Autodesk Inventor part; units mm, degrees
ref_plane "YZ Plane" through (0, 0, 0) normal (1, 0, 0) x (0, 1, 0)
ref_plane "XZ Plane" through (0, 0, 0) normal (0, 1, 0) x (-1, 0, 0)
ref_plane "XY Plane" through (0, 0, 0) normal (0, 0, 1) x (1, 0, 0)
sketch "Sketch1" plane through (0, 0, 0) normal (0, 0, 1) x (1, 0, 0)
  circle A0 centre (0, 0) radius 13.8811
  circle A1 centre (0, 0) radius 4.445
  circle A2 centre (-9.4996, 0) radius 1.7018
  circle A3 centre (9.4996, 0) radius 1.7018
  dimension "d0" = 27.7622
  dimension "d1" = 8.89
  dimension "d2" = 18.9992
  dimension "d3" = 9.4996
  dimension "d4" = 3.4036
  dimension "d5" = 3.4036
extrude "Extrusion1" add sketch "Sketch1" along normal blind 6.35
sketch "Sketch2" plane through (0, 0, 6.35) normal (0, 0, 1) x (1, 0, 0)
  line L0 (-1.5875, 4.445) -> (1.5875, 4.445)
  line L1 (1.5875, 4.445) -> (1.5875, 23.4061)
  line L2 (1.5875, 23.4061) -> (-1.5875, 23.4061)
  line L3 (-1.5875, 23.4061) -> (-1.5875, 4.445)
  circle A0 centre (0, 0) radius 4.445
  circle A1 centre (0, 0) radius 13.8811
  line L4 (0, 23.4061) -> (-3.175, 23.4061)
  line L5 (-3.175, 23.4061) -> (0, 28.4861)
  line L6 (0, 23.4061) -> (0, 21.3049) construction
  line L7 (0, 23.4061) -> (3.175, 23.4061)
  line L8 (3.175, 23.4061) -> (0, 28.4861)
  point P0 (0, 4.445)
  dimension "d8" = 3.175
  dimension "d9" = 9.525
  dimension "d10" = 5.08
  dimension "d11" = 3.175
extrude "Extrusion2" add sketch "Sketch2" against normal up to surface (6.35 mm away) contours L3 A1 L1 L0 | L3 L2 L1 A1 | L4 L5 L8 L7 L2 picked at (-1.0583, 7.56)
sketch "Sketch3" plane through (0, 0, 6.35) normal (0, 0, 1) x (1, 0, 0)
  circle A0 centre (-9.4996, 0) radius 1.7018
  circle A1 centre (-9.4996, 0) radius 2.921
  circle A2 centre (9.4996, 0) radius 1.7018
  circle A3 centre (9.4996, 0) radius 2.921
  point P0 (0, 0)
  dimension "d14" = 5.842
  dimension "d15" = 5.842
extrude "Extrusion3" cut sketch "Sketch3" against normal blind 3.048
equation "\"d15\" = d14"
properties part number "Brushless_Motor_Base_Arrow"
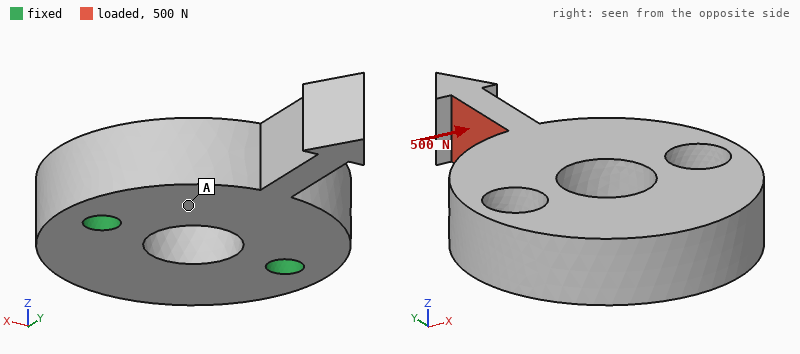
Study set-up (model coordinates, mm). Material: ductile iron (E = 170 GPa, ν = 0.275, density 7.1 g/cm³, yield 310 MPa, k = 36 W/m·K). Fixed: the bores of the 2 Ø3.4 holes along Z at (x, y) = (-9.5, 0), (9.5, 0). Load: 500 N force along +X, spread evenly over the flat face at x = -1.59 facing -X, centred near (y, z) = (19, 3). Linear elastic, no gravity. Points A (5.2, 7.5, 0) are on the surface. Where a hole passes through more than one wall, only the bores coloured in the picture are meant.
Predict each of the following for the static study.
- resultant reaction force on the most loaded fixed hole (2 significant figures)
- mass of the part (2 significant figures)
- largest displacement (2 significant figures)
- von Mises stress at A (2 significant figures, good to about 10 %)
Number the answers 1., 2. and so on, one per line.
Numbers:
1. 510 N
2. 25 g
3. 52 µm
4. 17 MPa
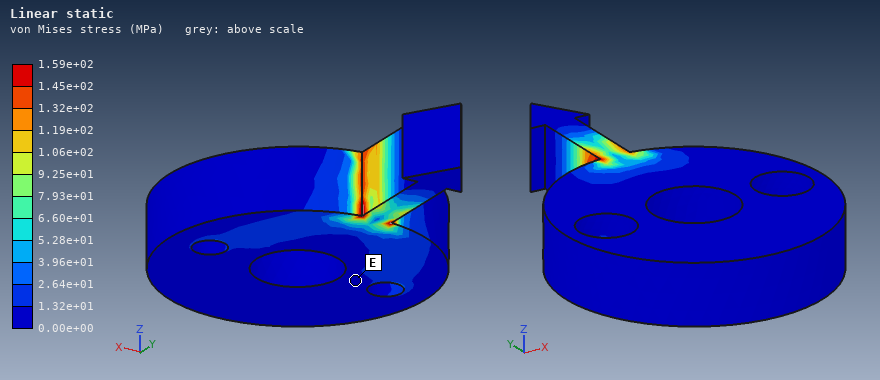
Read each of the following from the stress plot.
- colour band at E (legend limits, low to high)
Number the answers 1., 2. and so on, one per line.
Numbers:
1. 0.00e+00 to 1.32e+01 MPa
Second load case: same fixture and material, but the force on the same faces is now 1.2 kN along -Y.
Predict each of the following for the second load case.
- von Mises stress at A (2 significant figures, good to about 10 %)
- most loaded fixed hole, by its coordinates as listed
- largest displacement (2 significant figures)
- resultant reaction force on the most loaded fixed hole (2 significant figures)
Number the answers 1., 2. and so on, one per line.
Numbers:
1. 14 MPa
2. (-9.5, 0)
3. 48 µm
4. 740 N
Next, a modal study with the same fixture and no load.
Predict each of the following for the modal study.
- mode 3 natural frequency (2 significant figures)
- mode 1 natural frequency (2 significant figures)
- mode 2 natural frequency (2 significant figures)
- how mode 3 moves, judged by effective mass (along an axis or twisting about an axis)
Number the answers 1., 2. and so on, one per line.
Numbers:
1. 17 kHz
2. 8200 Hz
3. 10 kHz
4. along Z
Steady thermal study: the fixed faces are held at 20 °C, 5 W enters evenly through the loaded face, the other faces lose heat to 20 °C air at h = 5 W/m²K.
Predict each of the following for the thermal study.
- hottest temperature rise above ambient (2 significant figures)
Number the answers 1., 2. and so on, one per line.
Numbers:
1. 63 K
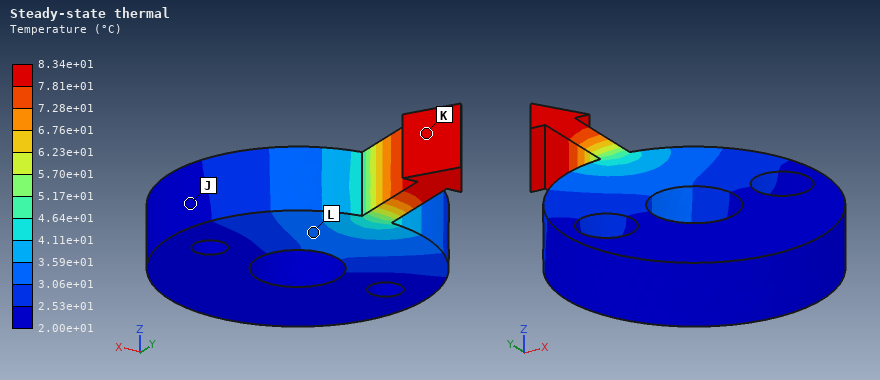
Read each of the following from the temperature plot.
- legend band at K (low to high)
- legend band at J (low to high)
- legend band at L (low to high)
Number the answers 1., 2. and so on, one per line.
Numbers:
1. 7.81e+01 to 8.34e+01 °C
2. 2.00e+01 to 2.53e+01 °C
3. 3.06e+01 to 3.59e+01 °C
